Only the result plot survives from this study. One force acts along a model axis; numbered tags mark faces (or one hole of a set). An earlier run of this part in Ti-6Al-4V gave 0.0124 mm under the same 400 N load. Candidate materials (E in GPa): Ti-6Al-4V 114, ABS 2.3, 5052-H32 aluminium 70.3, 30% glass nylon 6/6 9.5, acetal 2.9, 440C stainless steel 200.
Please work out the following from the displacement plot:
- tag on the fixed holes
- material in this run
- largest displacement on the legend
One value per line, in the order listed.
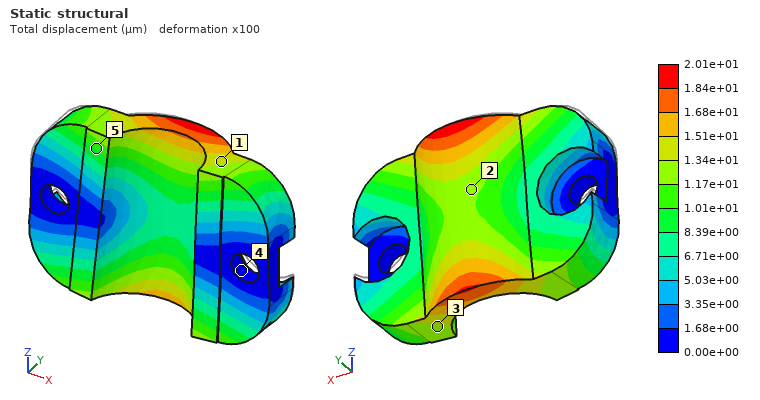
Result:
4
5052-H32 aluminium
2.01e+01 µm
